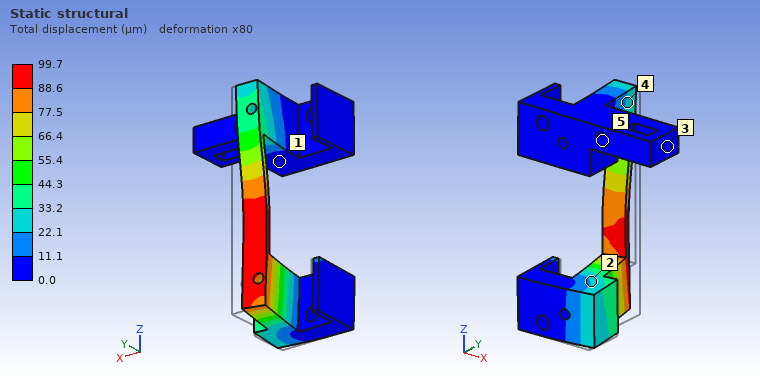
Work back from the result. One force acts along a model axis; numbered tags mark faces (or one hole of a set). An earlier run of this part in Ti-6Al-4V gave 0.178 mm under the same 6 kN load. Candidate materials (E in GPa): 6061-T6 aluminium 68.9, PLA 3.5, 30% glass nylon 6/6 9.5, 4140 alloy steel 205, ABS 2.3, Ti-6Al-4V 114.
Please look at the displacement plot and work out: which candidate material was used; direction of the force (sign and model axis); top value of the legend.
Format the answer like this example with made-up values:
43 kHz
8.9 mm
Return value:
4140 alloy steel
-X
99.7 µm
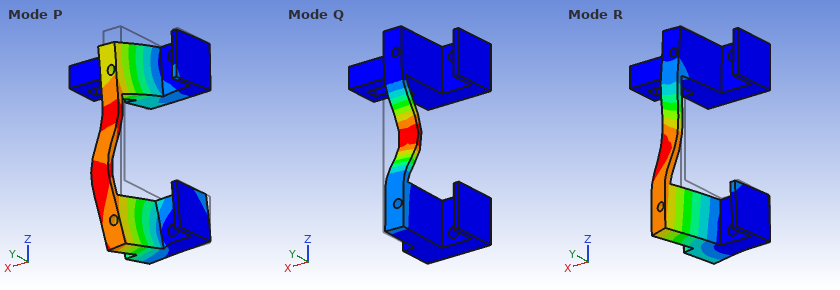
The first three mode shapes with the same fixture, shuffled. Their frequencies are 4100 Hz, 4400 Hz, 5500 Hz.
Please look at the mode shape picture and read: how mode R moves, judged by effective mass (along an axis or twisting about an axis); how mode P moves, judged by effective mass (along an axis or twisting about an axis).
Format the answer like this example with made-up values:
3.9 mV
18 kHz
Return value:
along X
along Z
